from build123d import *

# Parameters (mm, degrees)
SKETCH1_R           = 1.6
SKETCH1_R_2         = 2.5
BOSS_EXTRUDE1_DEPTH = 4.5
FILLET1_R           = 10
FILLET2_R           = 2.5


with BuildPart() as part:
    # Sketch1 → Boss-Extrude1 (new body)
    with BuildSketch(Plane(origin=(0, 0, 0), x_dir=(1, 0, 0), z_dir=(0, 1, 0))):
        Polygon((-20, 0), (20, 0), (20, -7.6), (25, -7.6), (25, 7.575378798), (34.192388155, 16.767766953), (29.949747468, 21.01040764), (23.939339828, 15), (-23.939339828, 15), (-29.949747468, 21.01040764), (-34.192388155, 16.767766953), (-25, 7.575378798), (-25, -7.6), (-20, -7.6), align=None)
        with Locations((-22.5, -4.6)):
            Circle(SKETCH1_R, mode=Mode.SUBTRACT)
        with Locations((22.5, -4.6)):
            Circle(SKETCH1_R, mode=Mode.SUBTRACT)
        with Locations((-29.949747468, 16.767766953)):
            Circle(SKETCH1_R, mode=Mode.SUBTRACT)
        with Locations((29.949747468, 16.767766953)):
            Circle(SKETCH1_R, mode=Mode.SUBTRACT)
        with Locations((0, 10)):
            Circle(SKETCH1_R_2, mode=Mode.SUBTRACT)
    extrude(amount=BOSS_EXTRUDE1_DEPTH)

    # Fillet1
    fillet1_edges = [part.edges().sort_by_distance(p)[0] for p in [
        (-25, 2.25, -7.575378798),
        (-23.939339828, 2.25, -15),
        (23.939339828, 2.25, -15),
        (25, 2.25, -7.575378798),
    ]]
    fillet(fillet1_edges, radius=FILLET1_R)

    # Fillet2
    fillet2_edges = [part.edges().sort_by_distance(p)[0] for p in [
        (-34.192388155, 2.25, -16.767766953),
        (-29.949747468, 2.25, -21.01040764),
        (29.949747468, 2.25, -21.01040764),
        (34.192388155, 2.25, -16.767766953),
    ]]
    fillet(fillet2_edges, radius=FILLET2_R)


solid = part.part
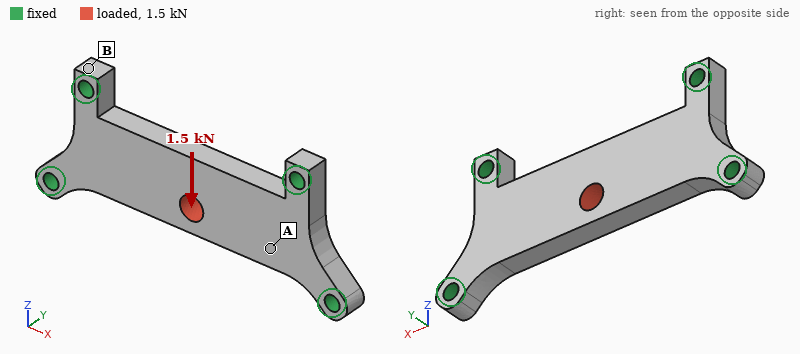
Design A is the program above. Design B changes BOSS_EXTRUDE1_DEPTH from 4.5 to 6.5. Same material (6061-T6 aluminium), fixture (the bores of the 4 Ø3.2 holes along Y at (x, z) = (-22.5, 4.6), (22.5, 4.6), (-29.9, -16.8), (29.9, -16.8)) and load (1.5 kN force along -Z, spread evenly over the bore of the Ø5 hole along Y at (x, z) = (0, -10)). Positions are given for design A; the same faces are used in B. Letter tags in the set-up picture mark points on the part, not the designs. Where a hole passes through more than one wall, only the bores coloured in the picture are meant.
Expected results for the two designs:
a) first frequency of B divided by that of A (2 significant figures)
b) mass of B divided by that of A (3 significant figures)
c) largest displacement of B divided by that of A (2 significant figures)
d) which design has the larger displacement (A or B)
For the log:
1.3
1.44
0.69
A
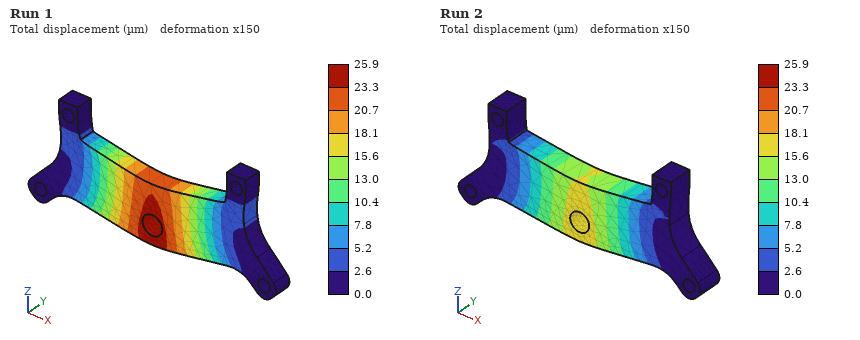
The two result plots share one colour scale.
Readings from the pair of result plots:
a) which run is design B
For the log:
Run 2
